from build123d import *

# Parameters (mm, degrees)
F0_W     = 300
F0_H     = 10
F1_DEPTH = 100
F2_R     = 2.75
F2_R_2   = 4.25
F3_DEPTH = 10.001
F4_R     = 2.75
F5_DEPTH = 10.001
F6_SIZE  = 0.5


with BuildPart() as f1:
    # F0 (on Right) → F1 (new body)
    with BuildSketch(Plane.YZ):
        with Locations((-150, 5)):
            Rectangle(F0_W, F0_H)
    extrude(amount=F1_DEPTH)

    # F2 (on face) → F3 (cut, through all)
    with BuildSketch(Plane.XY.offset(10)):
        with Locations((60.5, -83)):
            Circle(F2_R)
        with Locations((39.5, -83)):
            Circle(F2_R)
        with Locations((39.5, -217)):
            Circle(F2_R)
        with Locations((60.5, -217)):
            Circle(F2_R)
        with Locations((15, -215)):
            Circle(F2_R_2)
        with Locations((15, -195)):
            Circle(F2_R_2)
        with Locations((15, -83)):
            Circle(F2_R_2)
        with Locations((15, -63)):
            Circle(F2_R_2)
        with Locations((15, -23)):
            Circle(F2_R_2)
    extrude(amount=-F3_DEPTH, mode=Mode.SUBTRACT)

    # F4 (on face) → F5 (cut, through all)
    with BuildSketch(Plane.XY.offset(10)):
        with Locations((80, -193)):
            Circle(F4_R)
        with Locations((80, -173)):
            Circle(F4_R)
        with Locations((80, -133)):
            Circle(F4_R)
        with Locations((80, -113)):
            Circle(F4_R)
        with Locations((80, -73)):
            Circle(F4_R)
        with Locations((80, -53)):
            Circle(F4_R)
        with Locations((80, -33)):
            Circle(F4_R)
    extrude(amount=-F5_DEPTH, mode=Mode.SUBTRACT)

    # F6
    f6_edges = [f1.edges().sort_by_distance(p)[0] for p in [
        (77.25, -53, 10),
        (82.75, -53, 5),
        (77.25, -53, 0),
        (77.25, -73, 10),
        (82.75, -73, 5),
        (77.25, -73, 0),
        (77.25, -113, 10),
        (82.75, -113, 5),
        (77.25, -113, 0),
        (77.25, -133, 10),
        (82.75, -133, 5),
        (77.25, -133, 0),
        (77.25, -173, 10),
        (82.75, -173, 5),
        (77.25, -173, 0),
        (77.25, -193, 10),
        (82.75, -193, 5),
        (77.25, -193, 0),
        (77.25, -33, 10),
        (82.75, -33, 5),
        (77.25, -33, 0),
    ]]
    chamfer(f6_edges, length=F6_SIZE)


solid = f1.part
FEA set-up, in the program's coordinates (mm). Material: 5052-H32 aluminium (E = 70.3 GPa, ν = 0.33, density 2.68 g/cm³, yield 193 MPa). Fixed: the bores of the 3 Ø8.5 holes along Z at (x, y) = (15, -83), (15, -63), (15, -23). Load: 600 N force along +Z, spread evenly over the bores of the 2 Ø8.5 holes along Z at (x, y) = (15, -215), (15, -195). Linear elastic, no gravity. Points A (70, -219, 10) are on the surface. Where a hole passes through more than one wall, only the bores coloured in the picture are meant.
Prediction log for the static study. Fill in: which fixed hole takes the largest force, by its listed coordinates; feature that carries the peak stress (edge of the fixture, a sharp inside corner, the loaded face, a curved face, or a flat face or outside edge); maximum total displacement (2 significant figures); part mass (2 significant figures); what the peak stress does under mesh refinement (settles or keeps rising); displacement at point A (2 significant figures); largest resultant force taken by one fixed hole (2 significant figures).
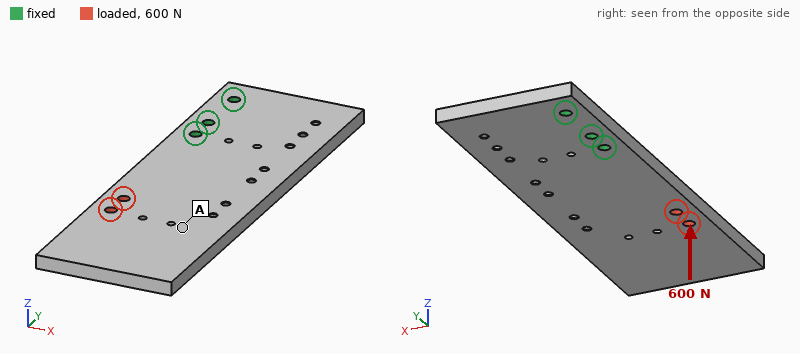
(15, -83)
edge of the fixture
1.7 mm
790 g
keeps rising
0.87 mm
1.7 kN
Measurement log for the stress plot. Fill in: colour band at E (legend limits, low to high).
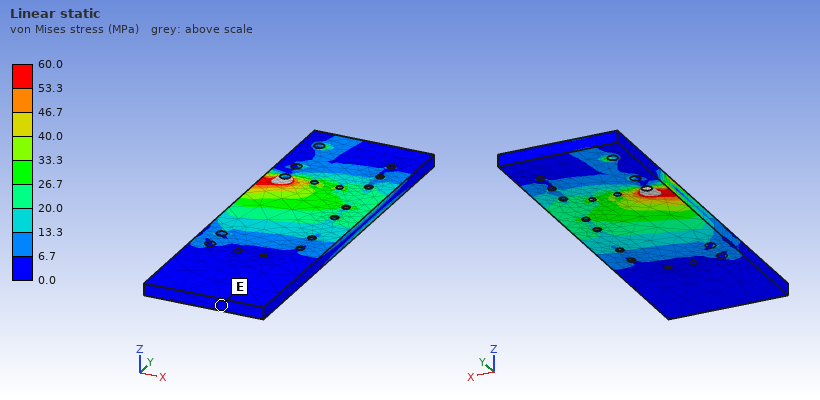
0.0 to 6.7 MPa
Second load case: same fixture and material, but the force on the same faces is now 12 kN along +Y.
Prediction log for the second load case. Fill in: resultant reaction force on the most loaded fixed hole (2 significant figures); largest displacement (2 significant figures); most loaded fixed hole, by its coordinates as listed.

9.1 kN
0.15 mm
(15, -83)
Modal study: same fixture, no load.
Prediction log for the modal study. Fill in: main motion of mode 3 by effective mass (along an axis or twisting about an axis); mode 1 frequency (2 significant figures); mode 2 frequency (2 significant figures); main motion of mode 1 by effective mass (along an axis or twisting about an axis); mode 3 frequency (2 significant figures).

along Z
160 Hz
600 Hz
along Z
970 Hz
